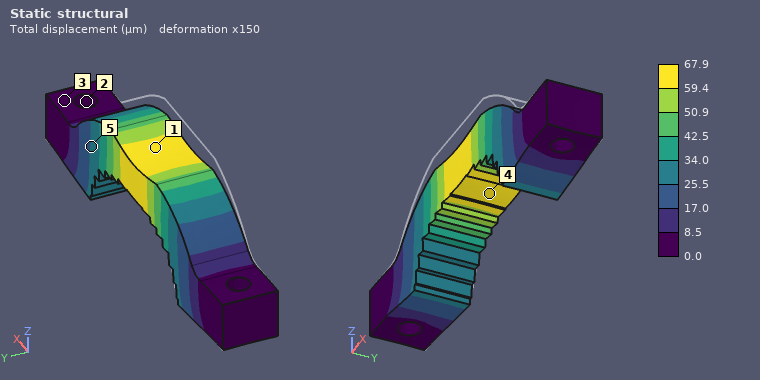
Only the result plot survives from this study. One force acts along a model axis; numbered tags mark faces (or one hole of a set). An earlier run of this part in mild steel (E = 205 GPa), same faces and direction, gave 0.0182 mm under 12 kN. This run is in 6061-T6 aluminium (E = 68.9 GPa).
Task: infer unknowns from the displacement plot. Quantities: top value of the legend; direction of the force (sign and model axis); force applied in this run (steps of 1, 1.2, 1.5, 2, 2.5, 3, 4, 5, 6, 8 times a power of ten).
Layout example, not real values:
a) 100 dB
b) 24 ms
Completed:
a) 67.9 µm
b) -Z
c) 15 kN
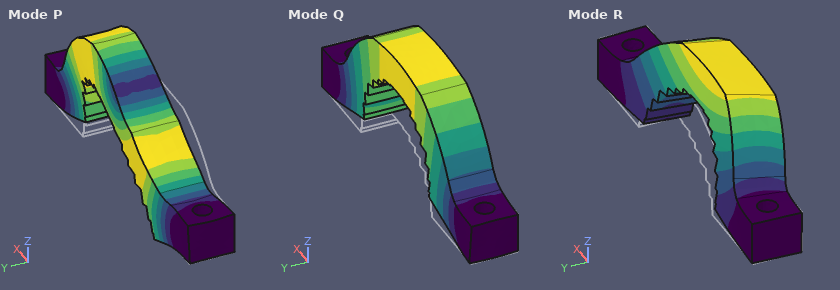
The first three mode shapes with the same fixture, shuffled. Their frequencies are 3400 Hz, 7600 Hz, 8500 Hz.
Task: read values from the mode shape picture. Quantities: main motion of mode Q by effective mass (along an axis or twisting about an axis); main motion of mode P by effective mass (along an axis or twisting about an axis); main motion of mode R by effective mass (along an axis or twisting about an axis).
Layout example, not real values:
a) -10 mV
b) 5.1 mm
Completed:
a) along Z
b) along X
c) along Y
